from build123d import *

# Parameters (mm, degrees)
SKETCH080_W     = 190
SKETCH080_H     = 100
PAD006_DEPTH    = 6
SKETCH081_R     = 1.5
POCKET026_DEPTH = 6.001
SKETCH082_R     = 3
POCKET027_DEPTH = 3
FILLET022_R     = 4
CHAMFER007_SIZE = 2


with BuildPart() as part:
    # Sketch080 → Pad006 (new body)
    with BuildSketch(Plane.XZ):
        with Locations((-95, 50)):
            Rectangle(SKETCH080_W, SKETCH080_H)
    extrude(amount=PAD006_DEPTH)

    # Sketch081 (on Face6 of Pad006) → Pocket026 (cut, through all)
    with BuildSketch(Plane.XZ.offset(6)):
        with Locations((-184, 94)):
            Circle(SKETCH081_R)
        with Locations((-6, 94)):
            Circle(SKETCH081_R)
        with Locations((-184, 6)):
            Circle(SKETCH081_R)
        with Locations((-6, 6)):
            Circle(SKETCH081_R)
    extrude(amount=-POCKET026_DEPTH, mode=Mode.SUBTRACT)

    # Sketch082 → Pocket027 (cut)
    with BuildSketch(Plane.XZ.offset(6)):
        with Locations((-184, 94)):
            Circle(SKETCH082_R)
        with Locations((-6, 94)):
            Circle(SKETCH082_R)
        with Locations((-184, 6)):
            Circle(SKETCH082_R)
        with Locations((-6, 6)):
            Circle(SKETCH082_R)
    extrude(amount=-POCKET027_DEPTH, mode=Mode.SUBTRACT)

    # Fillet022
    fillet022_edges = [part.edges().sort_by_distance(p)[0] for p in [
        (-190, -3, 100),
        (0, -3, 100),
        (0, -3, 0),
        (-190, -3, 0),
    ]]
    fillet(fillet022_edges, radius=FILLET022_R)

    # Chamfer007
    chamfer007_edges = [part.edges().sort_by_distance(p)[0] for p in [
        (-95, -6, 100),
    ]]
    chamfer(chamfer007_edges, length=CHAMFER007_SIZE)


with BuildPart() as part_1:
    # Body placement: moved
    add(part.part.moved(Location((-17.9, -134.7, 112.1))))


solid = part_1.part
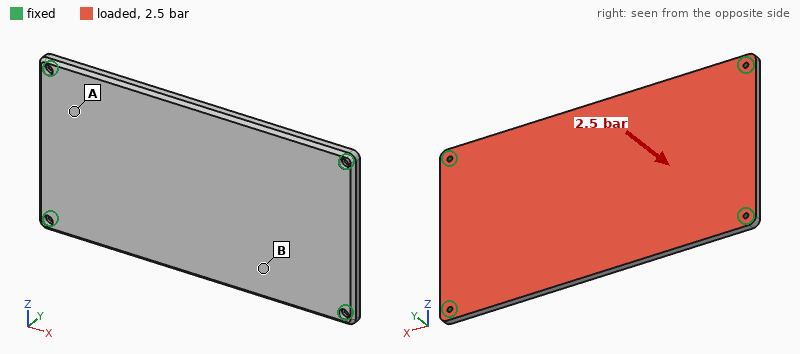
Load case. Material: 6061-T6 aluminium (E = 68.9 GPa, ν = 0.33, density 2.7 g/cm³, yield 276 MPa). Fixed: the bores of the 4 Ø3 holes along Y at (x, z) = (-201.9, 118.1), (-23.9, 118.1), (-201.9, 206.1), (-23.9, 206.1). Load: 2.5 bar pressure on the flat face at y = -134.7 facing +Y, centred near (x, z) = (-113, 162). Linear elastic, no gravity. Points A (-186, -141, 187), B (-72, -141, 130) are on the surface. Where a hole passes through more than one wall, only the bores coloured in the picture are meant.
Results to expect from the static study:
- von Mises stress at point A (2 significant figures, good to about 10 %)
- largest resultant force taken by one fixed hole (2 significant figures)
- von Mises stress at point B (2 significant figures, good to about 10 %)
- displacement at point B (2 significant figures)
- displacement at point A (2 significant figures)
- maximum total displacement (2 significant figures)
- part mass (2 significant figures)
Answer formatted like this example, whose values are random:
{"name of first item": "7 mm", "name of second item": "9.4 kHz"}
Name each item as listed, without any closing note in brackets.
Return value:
{"von Mises stress at point A": "34 MPa", "largest resultant force taken by one fixed hole": "3.0 kN", "von Mises stress at point B": "68 MPa", "displacement at point B": "0.89 mm", "displacement at point A": "0.34 mm", "maximum total displacement": "1.3 mm", "part mass": "300 g"}
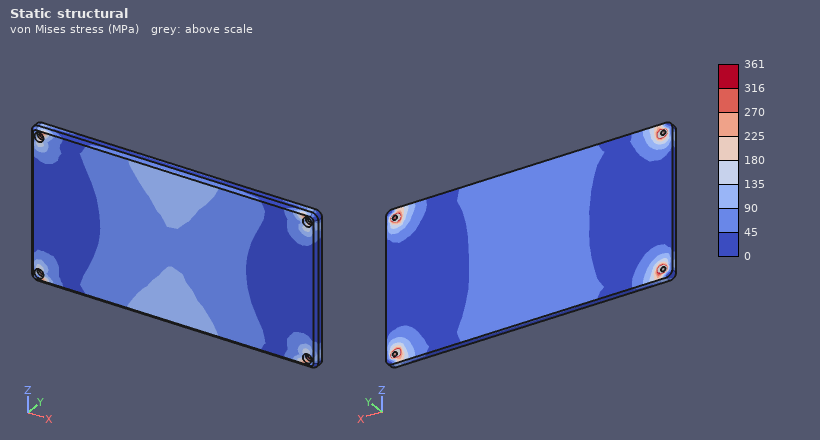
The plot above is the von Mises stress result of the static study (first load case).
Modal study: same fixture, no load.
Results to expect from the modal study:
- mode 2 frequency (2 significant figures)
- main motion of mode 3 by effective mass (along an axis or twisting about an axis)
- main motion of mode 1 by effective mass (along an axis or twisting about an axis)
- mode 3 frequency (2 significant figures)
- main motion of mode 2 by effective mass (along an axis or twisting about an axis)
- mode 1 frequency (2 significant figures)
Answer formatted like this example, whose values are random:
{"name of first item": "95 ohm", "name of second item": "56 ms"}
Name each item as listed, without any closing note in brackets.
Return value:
{"mode 2 frequency": "1300 Hz", "main motion of mode 3 by effective mass": "twisting about Z", "main motion of mode 1 by effective mass": "along Y", "mode 3 frequency": "1900 Hz", "main motion of mode 2 by effective mass": "twisting about X", "mode 1 frequency": "640 Hz"}
